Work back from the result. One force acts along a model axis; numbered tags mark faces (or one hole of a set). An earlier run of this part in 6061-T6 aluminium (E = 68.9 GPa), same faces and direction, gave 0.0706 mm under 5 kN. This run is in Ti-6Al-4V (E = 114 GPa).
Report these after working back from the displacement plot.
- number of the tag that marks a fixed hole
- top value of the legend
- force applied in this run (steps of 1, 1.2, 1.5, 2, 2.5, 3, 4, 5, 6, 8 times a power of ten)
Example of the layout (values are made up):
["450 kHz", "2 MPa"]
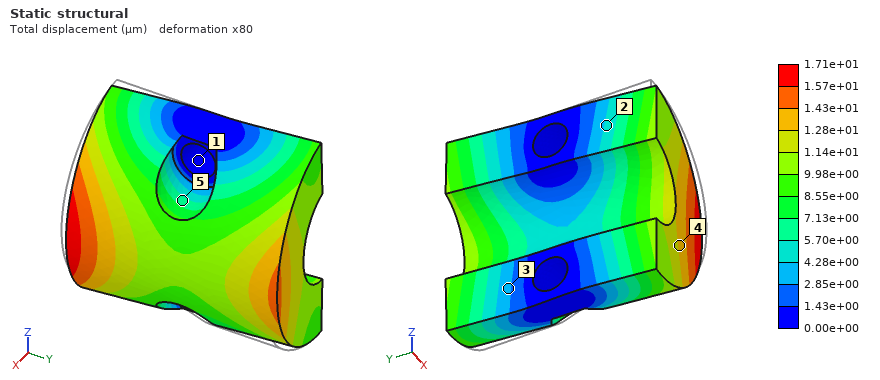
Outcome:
["1", "1.71e+01 µm", "2 kN"]
